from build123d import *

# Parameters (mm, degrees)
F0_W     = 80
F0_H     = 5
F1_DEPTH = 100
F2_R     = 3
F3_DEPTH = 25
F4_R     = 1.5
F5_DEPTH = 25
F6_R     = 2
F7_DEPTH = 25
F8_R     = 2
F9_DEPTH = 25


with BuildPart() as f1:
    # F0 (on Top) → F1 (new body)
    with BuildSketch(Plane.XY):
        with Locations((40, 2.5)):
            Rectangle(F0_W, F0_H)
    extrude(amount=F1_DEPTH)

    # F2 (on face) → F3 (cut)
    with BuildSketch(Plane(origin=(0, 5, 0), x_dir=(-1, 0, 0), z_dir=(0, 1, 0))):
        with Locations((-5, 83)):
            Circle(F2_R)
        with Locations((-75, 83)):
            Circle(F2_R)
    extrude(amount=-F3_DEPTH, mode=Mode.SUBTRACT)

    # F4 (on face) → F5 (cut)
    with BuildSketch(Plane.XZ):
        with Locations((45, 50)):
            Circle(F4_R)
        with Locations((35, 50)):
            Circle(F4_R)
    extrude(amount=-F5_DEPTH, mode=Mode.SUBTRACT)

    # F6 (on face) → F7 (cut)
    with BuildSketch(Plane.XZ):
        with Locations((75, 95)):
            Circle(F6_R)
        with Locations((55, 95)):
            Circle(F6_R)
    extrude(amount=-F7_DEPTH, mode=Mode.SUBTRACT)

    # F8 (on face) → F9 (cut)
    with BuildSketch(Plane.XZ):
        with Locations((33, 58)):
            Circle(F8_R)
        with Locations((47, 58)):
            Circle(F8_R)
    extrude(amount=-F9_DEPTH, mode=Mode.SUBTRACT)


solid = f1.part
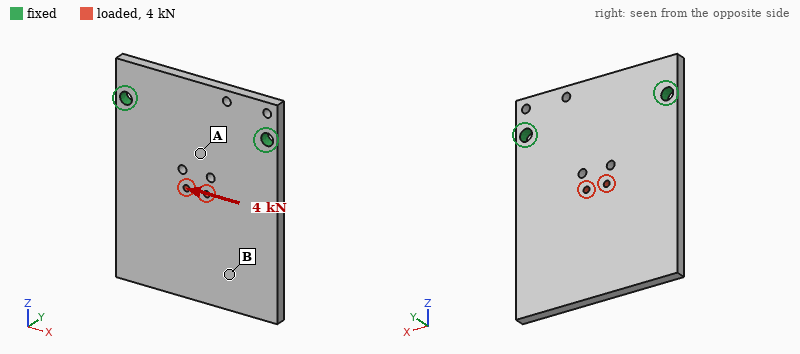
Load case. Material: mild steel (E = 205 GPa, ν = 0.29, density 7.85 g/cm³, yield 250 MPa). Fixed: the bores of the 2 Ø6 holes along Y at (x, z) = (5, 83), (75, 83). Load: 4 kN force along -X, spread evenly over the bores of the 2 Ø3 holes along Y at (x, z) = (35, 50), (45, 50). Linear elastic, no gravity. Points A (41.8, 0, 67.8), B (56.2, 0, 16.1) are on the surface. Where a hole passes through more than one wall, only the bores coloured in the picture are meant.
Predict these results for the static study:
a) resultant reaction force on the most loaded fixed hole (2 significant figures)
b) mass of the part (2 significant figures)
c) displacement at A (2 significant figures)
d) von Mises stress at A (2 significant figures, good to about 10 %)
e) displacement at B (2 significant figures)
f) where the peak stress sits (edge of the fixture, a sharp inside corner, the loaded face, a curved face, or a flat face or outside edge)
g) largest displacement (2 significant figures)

2.7 kN
310 g
3.4 µm
16 MPa
8.5 µm
the loaded face
9.4 µm
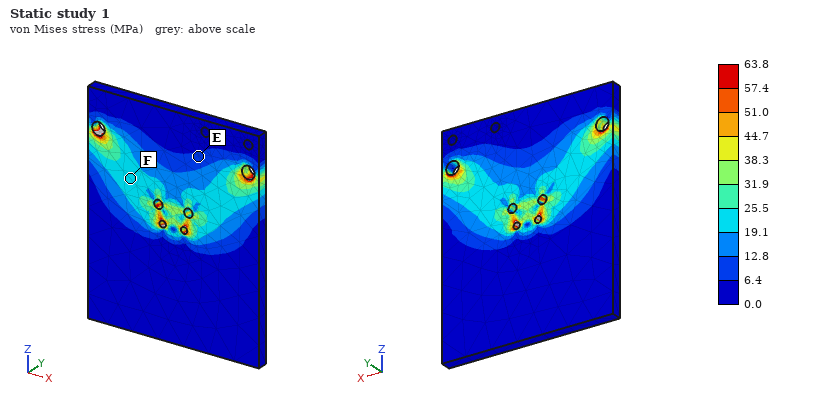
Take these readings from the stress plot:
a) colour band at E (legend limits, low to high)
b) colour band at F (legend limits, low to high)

6.4 to 12.8 MPa
19.1 to 25.5 MPa
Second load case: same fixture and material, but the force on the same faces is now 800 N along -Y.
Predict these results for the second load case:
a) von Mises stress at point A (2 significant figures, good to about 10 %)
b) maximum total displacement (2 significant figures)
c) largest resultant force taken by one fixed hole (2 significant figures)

42 MPa
0.28 mm
400 N
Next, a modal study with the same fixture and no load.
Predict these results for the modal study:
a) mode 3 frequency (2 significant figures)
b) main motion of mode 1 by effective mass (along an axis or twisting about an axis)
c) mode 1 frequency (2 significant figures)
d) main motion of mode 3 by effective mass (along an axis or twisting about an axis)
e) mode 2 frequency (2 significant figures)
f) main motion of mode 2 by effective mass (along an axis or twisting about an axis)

3300 Hz
along Y
530 Hz
along Y
1500 Hz
twisting about Z
